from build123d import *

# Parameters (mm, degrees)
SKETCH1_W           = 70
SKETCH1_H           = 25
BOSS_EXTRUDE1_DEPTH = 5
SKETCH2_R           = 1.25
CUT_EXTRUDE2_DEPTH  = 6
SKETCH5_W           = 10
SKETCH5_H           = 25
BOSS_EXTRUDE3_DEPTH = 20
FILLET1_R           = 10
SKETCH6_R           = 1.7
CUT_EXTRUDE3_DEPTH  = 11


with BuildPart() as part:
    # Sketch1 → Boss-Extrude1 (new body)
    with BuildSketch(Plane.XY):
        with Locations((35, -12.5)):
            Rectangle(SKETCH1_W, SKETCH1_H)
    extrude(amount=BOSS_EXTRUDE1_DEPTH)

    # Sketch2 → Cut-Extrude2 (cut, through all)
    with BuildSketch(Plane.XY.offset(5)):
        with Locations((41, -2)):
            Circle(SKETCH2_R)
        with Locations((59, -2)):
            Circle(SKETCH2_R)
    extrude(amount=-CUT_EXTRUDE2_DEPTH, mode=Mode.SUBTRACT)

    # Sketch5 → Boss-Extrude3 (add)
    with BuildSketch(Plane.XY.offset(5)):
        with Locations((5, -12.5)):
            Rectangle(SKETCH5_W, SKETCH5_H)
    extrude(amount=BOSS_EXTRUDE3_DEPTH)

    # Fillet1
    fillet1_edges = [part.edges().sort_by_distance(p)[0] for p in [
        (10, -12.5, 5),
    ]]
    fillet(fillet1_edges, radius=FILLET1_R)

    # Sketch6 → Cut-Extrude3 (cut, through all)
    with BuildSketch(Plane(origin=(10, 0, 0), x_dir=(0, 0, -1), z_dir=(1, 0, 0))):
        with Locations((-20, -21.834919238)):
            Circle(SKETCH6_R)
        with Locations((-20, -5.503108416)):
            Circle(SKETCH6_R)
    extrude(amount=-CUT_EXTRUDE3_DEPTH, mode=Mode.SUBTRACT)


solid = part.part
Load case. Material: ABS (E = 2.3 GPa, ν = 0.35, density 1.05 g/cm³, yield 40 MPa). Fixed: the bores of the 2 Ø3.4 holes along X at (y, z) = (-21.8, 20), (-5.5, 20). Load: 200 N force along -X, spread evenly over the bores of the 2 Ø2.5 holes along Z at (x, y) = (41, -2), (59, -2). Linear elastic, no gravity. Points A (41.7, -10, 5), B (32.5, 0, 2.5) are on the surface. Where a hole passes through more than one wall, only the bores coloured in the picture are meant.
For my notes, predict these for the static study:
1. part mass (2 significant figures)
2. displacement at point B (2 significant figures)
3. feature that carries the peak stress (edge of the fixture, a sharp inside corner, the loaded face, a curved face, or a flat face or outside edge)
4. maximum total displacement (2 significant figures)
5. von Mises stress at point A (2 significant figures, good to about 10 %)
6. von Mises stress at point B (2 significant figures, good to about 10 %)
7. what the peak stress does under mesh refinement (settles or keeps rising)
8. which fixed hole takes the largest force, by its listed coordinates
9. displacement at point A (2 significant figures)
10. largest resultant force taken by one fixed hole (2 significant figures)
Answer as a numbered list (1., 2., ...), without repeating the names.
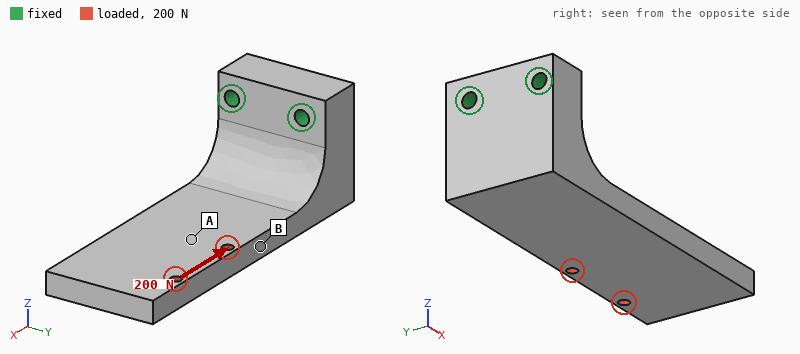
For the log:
1. 15 g
2. 0.34 mm
3. edge of the fixture
4. 0.76 mm
5. 1.8 MPa
6. 5.7 MPa
7. keeps rising
8. (-5.5, 20)
9. 0.37 mm
10. 210 N
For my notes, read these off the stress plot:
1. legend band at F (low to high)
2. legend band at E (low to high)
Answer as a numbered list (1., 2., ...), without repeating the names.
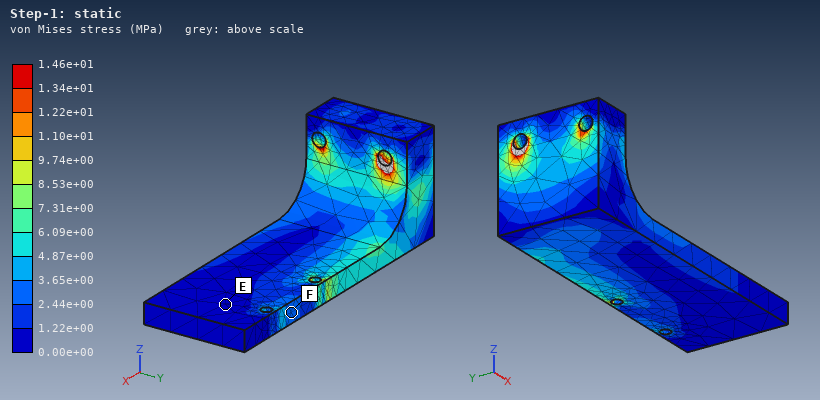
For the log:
1. 2.44e+00 to 3.65e+00 MPa
2. 0.00e+00 to 1.22e+00 MPa
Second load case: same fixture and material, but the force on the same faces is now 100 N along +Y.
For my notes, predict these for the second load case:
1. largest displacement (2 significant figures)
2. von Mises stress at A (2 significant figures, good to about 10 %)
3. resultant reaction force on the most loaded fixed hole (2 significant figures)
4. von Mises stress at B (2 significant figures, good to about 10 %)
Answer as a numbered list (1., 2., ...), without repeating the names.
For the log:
1. 0.83 mm
2. 1.7 MPa
3. 240 N
4. 3.5 MPa
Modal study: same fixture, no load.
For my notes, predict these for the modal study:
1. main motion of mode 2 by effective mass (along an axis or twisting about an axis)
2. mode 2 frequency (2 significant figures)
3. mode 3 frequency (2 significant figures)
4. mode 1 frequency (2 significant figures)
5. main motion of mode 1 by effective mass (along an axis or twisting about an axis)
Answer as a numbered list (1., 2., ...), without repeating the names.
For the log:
1. along Y
2. 880 Hz
3. 1600 Hz
4. 350 Hz
5. along Z
